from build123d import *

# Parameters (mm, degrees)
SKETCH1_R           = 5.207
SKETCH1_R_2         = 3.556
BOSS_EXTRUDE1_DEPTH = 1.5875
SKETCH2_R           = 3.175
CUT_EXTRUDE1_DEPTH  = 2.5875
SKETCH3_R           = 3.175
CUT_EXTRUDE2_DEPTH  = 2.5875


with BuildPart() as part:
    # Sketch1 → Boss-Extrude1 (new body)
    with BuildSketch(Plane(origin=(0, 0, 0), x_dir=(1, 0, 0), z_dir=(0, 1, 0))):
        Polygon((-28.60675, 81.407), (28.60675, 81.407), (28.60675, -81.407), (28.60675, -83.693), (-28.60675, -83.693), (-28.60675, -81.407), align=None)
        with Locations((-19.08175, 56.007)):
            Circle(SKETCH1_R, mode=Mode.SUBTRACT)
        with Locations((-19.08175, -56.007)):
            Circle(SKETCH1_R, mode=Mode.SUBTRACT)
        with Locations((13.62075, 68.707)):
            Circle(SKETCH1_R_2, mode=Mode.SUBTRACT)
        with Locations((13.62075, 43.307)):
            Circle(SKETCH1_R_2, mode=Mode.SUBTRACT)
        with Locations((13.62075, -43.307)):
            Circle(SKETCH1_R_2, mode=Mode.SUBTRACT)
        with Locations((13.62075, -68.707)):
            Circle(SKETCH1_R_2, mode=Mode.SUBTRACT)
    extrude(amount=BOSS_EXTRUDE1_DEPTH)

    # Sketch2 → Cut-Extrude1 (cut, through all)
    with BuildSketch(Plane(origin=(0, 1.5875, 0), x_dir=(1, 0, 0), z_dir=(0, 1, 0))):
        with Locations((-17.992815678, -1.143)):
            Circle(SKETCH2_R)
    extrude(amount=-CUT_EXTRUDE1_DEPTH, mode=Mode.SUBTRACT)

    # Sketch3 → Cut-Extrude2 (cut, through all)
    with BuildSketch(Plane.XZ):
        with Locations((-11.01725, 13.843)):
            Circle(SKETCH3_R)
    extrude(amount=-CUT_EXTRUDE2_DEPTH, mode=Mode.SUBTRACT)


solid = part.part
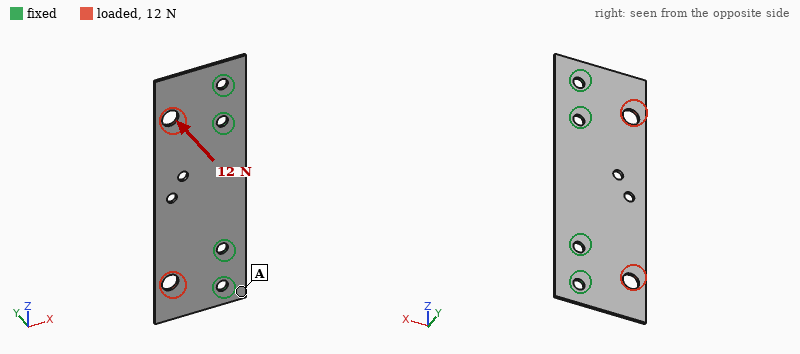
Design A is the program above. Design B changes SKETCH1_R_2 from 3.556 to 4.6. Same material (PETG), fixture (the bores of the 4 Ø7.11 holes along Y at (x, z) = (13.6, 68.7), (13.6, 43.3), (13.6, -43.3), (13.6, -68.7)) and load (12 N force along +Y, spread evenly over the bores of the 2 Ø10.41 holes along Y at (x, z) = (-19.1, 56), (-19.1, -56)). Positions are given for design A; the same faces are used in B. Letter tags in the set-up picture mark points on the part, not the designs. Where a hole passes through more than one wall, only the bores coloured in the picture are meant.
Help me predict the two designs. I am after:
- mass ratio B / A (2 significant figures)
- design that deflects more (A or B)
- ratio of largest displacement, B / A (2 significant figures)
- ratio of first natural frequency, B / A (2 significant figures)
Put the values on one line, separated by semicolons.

0.99; A; 0.90; 1.1
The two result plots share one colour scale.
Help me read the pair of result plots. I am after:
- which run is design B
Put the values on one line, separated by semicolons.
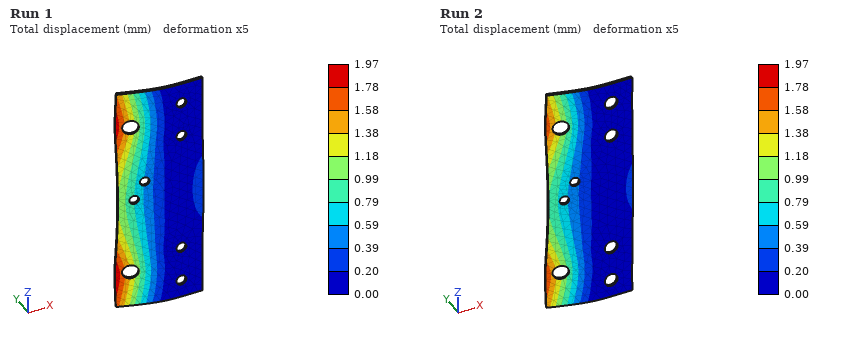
Run 2
